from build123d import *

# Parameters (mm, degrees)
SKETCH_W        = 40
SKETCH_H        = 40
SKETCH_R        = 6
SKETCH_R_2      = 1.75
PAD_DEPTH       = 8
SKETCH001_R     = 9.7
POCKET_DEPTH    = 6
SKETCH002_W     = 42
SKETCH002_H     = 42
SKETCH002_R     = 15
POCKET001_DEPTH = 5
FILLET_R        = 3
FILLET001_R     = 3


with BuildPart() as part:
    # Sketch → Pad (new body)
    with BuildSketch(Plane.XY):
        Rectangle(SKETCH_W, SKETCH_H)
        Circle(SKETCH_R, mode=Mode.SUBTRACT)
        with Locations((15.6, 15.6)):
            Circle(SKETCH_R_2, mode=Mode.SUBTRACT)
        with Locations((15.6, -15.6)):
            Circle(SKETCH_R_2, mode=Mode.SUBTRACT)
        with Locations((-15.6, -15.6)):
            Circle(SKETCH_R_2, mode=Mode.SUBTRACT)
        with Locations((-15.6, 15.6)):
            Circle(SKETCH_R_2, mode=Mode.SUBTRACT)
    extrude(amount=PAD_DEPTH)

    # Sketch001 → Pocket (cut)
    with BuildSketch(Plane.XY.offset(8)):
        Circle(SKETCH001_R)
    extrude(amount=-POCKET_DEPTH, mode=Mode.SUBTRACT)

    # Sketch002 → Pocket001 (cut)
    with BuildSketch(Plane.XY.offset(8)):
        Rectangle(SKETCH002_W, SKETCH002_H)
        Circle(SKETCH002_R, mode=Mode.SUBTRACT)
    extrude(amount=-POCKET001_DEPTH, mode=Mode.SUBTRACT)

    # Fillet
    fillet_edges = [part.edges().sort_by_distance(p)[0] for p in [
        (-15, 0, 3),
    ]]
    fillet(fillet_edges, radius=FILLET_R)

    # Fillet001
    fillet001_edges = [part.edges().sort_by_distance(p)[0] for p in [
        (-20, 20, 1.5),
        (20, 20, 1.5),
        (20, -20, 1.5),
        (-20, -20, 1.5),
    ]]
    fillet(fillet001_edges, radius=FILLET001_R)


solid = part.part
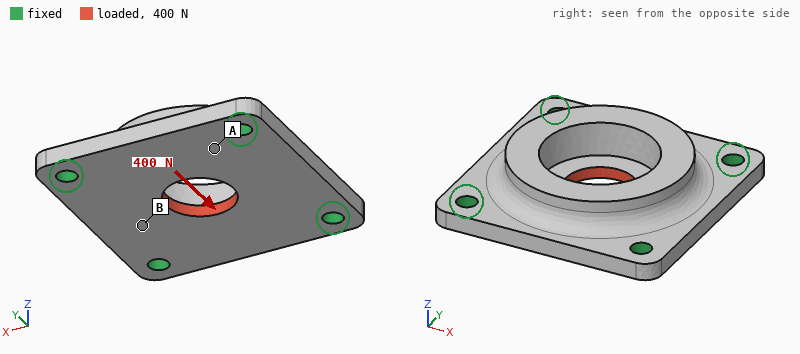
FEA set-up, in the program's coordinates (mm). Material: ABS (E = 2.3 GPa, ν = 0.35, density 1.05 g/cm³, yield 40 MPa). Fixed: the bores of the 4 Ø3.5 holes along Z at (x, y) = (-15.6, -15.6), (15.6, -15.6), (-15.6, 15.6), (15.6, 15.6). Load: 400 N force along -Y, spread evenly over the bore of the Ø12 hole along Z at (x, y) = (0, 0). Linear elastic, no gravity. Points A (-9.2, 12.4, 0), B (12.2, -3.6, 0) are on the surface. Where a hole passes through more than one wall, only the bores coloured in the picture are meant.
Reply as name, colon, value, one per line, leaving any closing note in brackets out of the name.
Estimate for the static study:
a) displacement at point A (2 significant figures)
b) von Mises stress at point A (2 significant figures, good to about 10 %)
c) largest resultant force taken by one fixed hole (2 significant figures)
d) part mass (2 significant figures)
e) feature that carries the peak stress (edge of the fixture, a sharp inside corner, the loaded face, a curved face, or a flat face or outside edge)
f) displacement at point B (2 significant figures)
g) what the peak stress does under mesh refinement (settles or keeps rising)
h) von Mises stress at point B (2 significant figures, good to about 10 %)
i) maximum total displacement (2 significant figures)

displacement at point A: 17 µm
von Mises stress at point A: 3.9 MPa
largest resultant force taken by one fixed hole: 110 N
part mass: 6.7 g
feature that carries the peak stress: edge of the fixture
displacement at point B: 14 µm
what the peak stress does under mesh refinement: keeps rising
von Mises stress at point B: 1.9 MPa
maximum total displacement: 43 µm
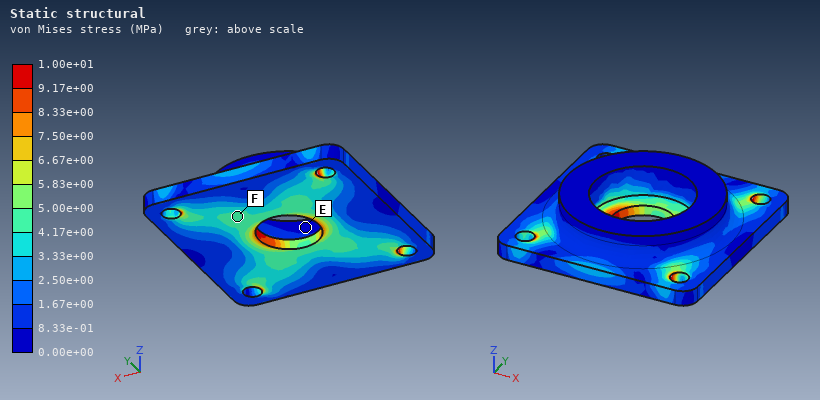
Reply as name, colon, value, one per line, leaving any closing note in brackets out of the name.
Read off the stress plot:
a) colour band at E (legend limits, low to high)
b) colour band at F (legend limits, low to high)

colour band at E: 0.00e+00 to 8.33e-01 MPa
colour band at F: 4.17e+00 to 5.00e+00 MPa
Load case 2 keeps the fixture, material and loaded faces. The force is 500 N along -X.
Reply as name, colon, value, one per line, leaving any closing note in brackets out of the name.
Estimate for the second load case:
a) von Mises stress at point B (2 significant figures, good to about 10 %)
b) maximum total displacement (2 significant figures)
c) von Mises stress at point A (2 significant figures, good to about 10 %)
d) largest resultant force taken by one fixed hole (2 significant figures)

von Mises stress at point B: 4.0 MPa
maximum total displacement: 54 µm
von Mises stress at point A: 4.2 MPa
largest resultant force taken by one fixed hole: 140 N
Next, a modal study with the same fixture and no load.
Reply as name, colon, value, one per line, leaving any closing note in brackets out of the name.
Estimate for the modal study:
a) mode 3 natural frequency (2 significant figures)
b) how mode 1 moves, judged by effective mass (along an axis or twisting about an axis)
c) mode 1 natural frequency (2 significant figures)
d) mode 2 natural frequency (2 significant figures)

mode 3 natural frequency: 6000 Hz
how mode 1 moves, judged by effective mass: along Z
mode 1 natural frequency: 4600 Hz
mode 2 natural frequency: 6000 Hz
